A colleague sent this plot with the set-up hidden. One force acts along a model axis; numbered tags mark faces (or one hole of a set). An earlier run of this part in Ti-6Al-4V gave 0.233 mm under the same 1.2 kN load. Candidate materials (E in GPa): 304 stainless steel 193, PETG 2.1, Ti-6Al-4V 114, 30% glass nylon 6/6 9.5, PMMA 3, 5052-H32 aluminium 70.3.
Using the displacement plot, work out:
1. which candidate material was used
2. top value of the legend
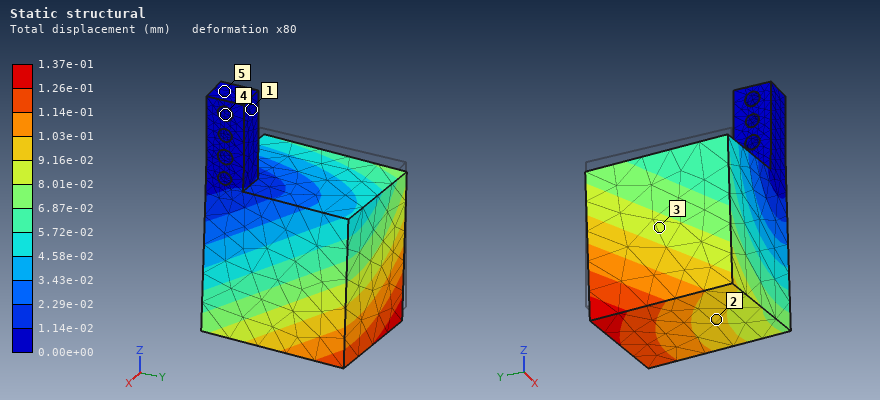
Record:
304 stainless steel
1.37e-01 mm
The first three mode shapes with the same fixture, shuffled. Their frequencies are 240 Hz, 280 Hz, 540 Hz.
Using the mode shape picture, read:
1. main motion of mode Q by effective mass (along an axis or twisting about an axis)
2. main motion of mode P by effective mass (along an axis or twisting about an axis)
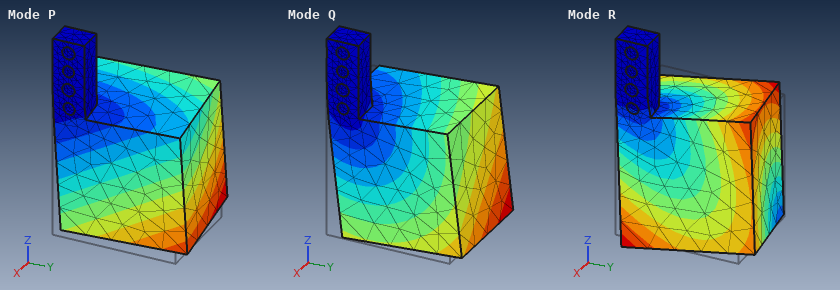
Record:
along Y
along X
